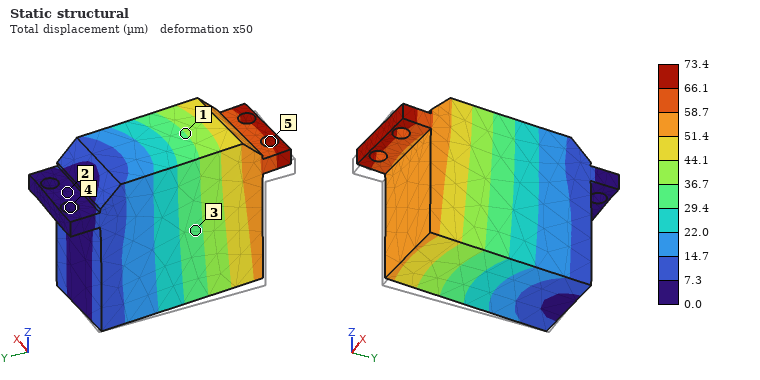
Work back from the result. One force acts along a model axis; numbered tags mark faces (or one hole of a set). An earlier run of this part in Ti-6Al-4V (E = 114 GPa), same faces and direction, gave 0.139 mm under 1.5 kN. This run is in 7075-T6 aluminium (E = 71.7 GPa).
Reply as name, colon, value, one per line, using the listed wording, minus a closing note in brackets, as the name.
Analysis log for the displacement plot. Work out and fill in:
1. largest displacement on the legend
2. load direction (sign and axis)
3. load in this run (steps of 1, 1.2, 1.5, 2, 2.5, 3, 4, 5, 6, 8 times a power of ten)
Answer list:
largest displacement on the legend: 73.4 µm
load direction: +X
load in this run: 500 N
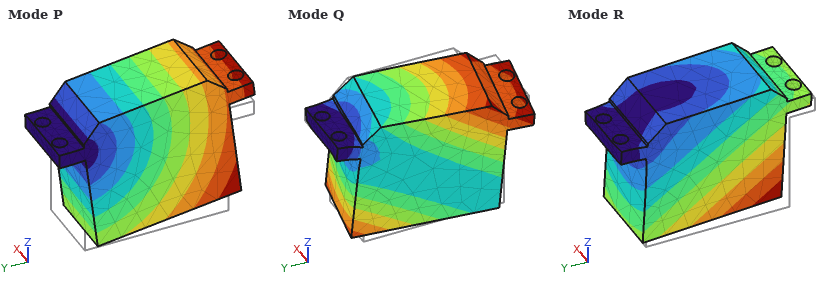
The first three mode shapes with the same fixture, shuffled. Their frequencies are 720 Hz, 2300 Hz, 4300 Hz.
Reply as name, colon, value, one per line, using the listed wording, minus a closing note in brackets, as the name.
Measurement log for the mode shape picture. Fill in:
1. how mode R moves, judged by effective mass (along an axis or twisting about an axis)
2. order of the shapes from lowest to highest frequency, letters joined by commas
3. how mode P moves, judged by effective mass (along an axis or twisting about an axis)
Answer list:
how mode R moves, judged by effective mass: along X
order of the shapes from lowest to highest frequency, letters joined by commas: P, R, Q
how mode P moves, judged by effective mass: along Z
